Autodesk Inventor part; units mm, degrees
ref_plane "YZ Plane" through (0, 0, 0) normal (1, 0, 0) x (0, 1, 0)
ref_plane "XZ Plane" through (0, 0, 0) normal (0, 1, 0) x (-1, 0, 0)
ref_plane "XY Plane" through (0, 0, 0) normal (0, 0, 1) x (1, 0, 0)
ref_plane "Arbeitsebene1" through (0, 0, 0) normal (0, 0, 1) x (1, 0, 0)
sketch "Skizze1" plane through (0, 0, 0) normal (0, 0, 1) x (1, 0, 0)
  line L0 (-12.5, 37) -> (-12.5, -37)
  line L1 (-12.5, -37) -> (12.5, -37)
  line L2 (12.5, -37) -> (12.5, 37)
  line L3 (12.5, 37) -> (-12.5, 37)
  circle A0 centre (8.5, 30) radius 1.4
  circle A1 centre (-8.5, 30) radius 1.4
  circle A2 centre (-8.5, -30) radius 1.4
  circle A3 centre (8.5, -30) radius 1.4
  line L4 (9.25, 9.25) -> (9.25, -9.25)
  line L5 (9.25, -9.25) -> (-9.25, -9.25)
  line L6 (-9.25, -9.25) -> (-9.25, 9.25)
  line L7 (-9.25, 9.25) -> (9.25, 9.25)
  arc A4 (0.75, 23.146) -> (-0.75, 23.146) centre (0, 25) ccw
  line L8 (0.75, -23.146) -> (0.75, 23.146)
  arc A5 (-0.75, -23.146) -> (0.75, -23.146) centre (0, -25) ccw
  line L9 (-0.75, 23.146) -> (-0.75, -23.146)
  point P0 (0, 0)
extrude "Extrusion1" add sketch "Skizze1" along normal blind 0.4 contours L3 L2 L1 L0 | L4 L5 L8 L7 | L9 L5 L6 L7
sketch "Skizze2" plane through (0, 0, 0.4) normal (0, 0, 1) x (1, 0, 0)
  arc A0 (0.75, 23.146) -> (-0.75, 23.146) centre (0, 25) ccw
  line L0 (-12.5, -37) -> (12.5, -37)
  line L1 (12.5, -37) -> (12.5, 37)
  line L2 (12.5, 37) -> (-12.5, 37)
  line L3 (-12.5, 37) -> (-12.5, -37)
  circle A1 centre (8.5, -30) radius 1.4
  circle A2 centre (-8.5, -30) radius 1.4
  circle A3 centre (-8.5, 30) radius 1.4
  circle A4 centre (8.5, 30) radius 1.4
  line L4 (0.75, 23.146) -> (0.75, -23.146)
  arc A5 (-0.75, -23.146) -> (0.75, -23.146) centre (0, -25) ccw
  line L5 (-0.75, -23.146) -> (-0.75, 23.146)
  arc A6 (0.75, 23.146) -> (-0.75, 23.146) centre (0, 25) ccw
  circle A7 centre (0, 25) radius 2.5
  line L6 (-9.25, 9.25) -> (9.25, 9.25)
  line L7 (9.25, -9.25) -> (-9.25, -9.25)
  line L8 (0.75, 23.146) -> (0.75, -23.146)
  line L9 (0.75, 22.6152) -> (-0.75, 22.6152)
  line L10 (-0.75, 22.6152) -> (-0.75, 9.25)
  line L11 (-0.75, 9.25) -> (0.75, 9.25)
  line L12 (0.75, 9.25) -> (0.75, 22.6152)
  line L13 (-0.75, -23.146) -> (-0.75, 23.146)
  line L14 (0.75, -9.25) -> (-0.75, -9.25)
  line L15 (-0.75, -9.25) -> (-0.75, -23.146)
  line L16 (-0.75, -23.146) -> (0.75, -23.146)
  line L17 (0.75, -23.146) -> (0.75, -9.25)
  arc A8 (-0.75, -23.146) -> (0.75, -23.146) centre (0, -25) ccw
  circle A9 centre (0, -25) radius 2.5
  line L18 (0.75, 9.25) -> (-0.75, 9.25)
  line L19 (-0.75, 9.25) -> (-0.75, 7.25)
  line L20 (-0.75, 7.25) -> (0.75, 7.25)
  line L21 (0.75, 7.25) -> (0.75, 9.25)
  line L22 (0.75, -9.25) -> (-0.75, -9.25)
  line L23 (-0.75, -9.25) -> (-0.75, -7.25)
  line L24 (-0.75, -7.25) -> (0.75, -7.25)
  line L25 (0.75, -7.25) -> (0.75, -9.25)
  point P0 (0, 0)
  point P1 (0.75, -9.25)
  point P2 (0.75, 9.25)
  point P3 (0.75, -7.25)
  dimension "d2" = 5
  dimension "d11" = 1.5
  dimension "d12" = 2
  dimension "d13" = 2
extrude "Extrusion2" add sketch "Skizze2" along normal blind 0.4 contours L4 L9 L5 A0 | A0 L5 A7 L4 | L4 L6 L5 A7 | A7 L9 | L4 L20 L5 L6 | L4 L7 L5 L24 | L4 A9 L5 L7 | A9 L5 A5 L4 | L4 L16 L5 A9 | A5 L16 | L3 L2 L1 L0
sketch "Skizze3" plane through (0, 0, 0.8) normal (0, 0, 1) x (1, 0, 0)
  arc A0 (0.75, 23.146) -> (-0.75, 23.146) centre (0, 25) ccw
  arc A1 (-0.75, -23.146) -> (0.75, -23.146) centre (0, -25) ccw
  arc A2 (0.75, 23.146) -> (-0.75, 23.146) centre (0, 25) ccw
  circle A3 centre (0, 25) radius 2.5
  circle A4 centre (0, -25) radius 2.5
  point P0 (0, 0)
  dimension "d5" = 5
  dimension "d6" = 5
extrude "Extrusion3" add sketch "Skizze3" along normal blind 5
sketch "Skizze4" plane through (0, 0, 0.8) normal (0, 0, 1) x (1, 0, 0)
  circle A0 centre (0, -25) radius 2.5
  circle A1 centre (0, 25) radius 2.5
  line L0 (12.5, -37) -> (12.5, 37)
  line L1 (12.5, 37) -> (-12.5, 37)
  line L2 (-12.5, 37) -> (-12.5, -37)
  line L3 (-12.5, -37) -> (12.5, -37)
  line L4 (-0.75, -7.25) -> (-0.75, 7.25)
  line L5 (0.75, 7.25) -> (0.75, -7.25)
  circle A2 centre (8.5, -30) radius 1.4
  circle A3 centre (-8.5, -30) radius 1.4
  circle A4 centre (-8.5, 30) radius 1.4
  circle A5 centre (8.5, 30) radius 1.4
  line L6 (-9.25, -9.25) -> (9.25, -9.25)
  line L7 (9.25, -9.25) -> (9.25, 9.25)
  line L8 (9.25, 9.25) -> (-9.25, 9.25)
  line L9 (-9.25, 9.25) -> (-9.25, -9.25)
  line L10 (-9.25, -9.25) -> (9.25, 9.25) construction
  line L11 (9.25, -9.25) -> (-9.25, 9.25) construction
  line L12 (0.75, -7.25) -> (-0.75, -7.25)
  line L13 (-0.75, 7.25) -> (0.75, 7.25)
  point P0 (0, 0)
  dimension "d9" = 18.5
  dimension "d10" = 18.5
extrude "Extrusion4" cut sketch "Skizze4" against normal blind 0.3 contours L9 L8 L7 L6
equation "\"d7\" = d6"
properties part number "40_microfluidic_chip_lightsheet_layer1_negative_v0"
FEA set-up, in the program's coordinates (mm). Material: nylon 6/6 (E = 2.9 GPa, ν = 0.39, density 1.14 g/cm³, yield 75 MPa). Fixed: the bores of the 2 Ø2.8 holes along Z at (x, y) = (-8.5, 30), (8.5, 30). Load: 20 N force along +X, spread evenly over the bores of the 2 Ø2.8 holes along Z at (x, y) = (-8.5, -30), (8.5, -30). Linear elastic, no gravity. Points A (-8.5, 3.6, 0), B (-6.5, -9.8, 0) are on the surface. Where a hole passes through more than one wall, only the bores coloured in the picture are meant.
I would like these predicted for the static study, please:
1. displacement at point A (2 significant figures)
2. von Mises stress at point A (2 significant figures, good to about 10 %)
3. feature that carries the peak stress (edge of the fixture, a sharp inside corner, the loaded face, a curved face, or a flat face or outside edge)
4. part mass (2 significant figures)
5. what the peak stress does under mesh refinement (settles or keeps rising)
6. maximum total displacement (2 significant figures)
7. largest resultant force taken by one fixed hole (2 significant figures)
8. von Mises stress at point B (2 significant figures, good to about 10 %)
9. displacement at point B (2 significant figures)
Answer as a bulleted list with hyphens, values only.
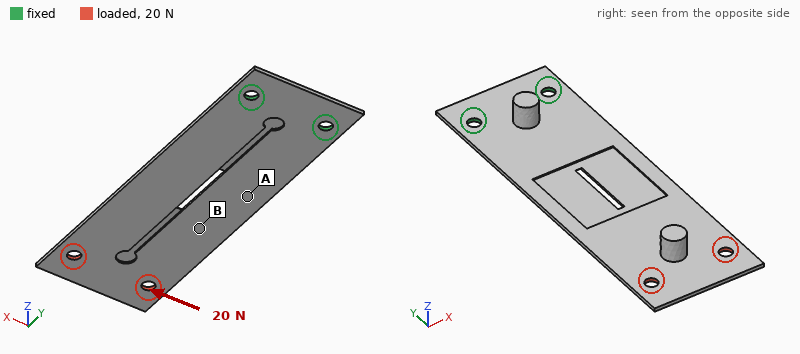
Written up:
- 0.22 mm
- 7.7 MPa
- a sharp inside corner
- 1.7 g
- keeps rising
- 0.83 mm
- 67 N
- 3.6 MPa
- 0.42 mm
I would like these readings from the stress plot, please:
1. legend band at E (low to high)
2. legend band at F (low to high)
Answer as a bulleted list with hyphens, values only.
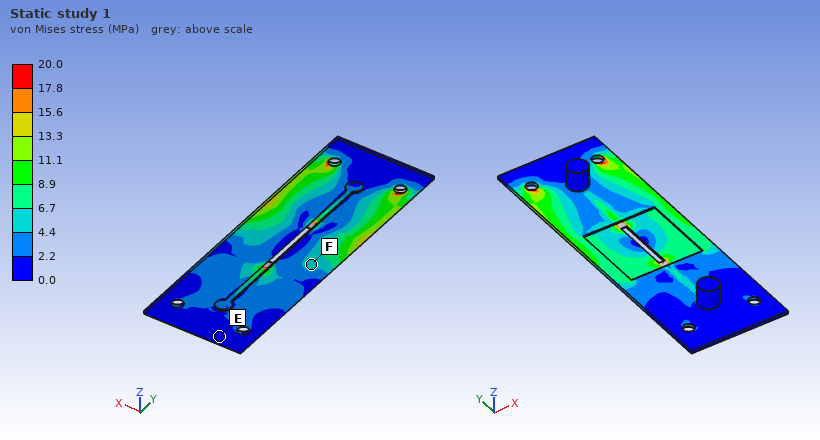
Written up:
- 0.0 to 2.2 MPa
- 4.4 to 6.7 MPa
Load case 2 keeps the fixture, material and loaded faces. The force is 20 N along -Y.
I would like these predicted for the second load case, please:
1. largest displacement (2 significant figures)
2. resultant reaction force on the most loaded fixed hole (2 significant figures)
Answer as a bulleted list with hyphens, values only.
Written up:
- 0.93 mm
- 10 N
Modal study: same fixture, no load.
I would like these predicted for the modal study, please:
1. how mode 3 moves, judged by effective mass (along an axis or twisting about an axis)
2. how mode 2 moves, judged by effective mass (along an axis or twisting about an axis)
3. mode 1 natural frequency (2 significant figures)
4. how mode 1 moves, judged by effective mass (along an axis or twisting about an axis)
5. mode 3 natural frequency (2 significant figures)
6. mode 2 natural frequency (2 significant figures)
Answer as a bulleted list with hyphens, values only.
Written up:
- along Z
- twisting about Y
- 41 Hz
- along Z
- 280 Hz
- 220 Hz
